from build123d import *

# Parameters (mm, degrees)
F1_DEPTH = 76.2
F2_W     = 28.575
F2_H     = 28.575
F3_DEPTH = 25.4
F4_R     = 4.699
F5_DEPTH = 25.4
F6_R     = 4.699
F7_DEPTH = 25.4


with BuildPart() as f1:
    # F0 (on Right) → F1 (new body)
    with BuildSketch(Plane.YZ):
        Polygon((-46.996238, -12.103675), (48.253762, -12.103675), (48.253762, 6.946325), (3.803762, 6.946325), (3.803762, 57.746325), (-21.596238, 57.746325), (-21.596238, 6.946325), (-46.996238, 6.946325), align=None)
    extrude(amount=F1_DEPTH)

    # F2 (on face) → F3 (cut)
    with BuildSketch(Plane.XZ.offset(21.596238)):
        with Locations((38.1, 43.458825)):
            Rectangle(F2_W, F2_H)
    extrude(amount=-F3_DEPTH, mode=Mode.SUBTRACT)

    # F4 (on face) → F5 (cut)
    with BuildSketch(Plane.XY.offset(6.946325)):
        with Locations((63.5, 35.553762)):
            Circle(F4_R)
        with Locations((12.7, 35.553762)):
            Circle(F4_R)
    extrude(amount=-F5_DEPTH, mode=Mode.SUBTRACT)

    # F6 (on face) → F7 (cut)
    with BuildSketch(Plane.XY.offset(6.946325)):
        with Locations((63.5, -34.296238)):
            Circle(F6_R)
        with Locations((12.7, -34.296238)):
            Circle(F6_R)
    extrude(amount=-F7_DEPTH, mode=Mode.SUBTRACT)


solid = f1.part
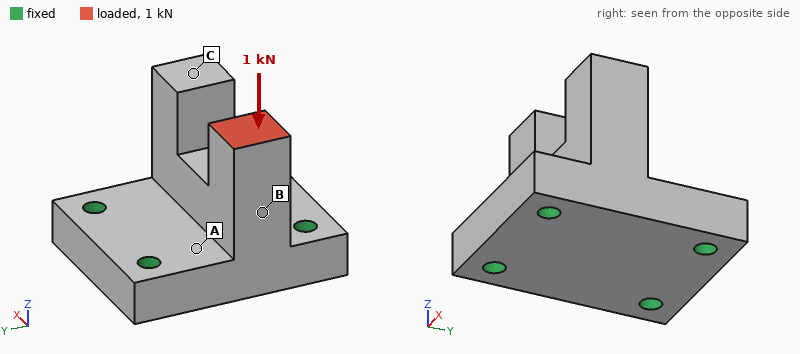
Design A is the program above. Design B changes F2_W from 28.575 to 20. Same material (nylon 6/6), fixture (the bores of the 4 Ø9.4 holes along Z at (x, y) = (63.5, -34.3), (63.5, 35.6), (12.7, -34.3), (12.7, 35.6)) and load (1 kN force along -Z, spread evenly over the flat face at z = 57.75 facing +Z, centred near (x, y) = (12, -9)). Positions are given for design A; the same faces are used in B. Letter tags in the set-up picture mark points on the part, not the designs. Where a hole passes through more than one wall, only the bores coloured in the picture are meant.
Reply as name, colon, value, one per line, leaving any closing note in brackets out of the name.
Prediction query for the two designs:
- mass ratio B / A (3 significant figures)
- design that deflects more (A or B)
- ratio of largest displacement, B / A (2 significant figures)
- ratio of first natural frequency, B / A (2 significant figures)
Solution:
mass ratio B / A: 1.03
design that deflects more: A
ratio of largest displacement, B / A: 0.89
ratio of first natural frequency, B / A: 0.95
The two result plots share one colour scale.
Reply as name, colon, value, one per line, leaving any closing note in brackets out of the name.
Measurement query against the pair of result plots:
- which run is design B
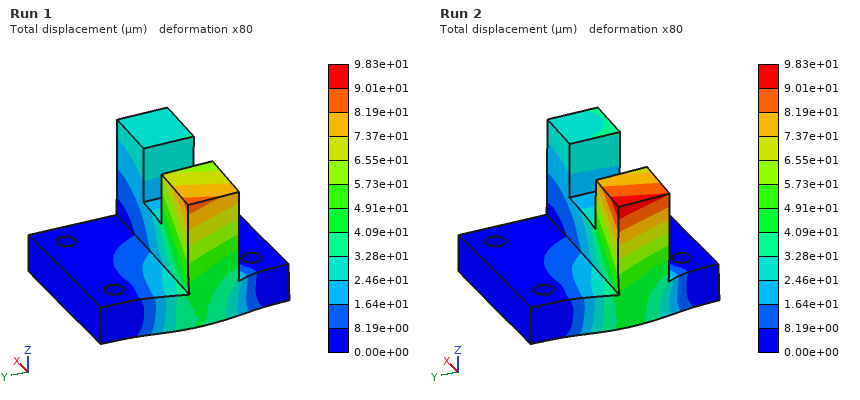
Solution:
which run is design B: Run 1
